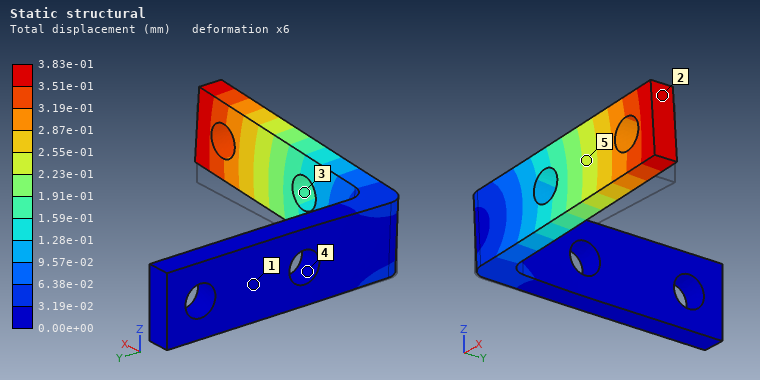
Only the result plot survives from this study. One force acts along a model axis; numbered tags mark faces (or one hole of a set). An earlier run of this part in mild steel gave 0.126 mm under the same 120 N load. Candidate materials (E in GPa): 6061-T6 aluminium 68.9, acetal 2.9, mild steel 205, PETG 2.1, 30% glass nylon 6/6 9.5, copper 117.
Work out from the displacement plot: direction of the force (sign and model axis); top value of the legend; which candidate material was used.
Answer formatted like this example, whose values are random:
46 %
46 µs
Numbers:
+Z
3.83e-01 mm
6061-T6 aluminium
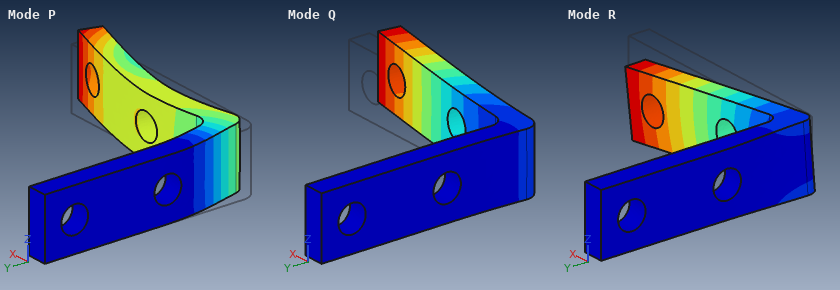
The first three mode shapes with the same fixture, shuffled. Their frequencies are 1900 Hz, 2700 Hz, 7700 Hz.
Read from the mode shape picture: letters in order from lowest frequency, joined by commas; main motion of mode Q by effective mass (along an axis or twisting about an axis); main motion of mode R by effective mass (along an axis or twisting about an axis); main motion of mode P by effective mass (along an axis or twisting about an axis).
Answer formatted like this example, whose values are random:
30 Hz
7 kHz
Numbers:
Q, R, P
along Y
along Z
along X
